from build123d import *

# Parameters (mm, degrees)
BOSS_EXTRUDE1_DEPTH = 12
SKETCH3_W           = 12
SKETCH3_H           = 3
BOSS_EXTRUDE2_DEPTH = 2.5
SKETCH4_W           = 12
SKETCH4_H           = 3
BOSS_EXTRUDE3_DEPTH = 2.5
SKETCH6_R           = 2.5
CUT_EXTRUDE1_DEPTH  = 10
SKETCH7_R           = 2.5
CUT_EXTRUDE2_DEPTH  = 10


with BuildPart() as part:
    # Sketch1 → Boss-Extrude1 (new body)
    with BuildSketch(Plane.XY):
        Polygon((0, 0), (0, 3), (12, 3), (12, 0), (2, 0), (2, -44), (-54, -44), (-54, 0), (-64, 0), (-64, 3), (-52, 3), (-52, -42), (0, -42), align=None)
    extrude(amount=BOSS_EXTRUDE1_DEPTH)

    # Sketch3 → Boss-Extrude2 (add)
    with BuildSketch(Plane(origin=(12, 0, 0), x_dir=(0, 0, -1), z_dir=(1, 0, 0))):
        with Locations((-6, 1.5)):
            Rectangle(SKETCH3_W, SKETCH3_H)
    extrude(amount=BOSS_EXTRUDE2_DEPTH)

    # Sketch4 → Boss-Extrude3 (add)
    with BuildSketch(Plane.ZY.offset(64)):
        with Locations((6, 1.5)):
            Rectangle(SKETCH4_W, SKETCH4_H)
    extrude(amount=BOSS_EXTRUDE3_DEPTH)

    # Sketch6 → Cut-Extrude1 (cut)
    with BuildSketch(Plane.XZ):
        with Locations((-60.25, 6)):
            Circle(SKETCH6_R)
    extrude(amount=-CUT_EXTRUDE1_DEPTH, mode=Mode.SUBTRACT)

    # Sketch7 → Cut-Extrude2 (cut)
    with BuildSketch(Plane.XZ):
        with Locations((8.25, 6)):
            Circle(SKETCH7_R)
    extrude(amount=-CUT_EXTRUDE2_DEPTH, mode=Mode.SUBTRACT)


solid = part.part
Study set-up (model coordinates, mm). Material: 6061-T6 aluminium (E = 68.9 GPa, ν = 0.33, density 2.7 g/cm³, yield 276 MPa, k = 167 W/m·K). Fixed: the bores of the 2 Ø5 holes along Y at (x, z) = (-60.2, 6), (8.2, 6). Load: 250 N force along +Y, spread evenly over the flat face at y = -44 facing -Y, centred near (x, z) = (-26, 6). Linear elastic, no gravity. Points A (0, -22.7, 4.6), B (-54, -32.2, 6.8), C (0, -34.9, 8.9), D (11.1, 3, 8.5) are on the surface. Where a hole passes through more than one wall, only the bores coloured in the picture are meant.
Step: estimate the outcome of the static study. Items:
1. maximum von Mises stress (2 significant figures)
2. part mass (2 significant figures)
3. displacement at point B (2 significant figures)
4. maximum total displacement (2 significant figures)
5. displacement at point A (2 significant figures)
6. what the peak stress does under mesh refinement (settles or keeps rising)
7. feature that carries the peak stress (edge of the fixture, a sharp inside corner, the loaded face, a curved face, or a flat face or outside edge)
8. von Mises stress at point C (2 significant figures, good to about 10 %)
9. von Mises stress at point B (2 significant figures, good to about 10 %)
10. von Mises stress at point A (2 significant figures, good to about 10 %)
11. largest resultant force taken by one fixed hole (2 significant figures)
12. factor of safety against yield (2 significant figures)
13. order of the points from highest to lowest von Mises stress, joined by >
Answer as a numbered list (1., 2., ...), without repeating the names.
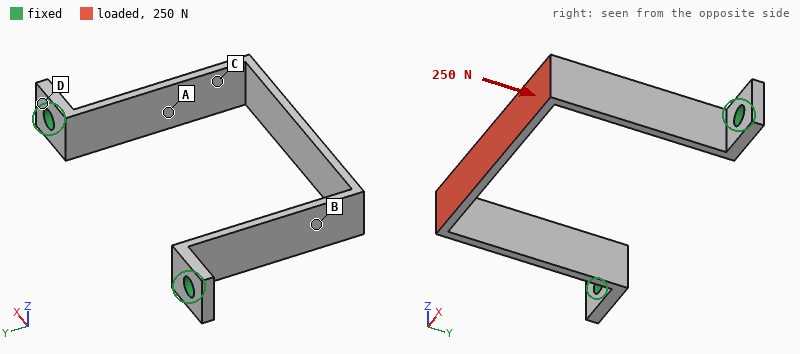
1. 100 MPa
2. 12 g
3. 0.094 mm
4. 0.38 mm
5. 0.090 mm
6. settles
7. the loaded face
8. 75 MPa
9. 55 MPa
10. 35 MPa
11. 130 N
12. 2.6
13. C > B > A > D
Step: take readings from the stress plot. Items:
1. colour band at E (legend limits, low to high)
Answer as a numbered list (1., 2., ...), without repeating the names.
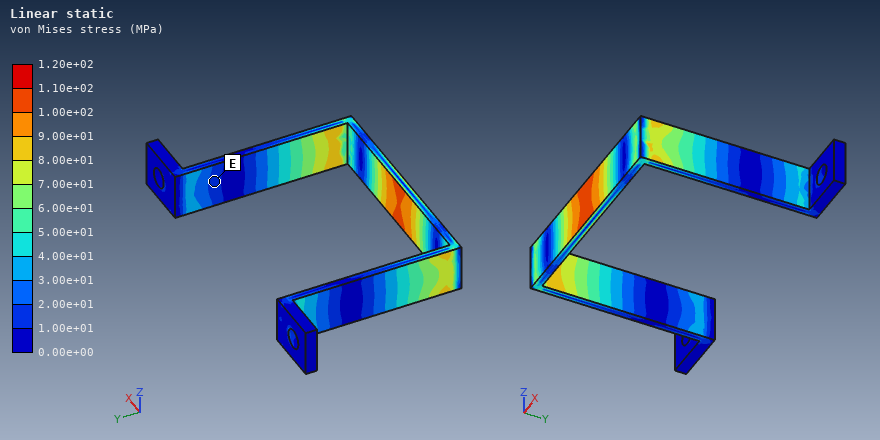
1. 1.00e+01 to 2.00e+01 MPa
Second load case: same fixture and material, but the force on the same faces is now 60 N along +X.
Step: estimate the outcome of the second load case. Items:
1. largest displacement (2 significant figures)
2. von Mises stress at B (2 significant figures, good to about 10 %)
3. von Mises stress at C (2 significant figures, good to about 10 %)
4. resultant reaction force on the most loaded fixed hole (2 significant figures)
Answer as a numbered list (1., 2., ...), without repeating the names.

1. 0.60 mm
2. 29 MPa
3. 41 MPa
4. 37 N
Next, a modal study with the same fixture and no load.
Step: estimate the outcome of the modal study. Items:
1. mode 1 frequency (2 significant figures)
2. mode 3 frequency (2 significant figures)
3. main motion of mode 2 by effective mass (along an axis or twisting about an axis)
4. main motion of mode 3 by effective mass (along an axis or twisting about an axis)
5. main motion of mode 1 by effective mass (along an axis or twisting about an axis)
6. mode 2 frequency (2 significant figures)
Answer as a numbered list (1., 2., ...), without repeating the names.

1. 690 Hz
2. 2000 Hz
3. along Z
4. twisting about Y
5. along X
6. 1400 Hz
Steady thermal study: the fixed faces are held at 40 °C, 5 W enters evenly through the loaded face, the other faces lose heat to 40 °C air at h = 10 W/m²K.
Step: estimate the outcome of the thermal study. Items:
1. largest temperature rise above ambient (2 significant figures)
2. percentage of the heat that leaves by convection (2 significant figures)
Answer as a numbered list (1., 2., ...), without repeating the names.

1. 34 K
2. 12 %
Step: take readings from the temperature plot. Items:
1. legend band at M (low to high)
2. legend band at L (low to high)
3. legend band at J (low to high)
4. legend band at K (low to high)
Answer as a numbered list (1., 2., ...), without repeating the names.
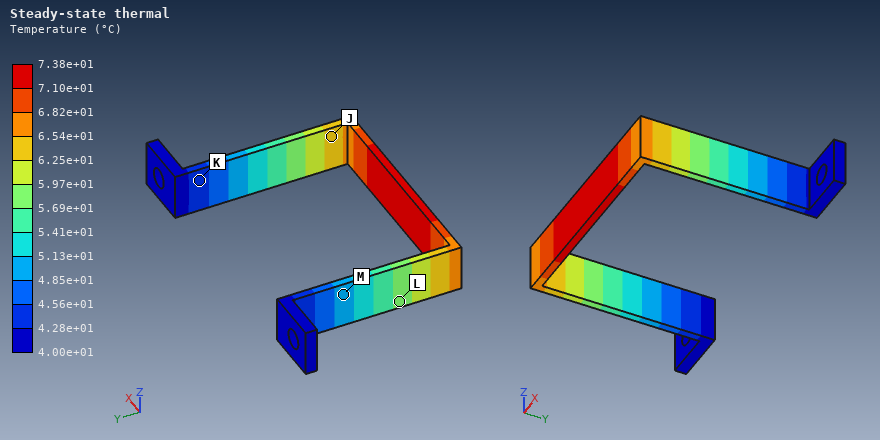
1. 4.85e+01 to 5.13e+01 °C
2. 5.69e+01 to 5.97e+01 °C
3. 6.25e+01 to 6.54e+01 °C
4. 4.28e+01 to 4.56e+01 °C
